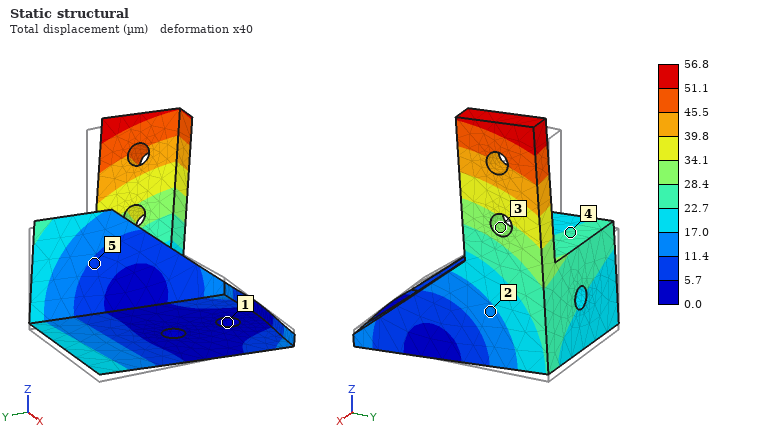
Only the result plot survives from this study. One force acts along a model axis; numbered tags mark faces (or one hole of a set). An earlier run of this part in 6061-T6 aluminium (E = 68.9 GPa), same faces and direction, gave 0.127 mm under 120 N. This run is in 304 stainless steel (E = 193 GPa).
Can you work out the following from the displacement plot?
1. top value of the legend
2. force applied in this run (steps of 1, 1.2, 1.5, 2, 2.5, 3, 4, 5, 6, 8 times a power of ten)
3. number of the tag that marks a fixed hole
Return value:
56.8 µm
150 N
1
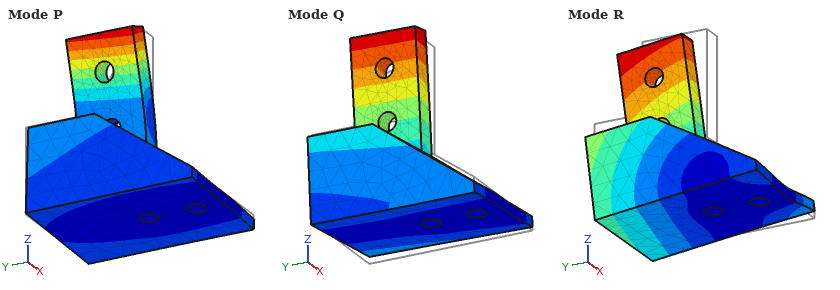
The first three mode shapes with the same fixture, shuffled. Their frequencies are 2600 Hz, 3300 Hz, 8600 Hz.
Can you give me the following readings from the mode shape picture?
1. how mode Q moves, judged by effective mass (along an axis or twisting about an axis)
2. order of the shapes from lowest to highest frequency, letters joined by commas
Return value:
along X
Q, R, P
